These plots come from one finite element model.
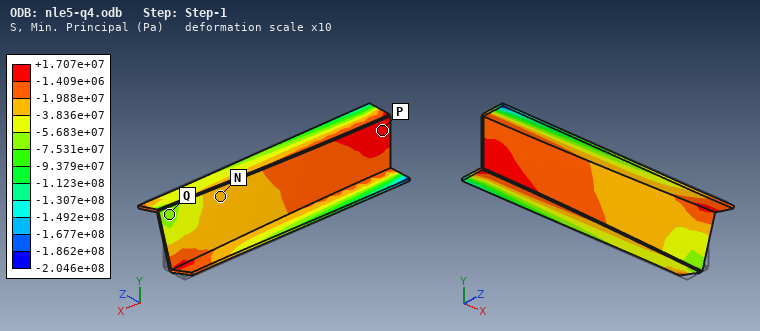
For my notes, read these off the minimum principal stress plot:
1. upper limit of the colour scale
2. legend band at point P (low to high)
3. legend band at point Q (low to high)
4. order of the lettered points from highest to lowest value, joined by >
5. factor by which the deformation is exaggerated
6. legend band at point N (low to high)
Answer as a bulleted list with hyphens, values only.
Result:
- +1.707e+07 Pa
- -1.409e+06 to +1.707e+07 Pa
- -7.531e+07 to -5.683e+07 Pa
- P > N > Q
- 10
- -3.836e+07 to -1.988e+07 Pa
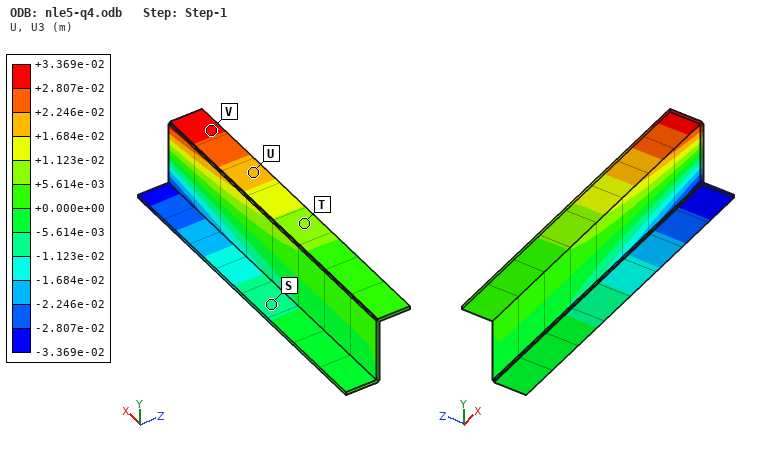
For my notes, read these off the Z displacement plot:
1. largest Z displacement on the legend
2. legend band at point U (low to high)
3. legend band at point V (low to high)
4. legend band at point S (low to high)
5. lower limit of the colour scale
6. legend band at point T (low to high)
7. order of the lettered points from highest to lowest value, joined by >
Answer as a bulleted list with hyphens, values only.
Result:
- +3.369e-02 m
- +1.684e-02 to +2.246e-02 m
- +2.807e-02 to +3.369e-02 m
- -1.123e-02 to -5.614e-03 m
- -3.369e-02 m
- +5.614e-03 to +1.123e-02 m
- V > U > T > S
